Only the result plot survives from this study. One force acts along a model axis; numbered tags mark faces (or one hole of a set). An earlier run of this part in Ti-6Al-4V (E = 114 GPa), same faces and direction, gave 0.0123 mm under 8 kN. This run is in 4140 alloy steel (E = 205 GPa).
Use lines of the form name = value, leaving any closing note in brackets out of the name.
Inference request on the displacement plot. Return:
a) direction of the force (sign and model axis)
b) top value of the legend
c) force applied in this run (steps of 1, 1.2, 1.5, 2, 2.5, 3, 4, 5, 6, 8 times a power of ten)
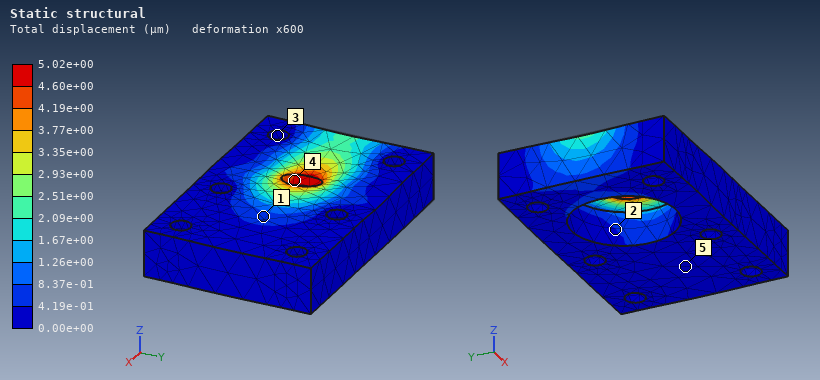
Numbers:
direction of the force = +X
top value of the legend = 5.02e+00 µm
force applied in this run = 6 kN
